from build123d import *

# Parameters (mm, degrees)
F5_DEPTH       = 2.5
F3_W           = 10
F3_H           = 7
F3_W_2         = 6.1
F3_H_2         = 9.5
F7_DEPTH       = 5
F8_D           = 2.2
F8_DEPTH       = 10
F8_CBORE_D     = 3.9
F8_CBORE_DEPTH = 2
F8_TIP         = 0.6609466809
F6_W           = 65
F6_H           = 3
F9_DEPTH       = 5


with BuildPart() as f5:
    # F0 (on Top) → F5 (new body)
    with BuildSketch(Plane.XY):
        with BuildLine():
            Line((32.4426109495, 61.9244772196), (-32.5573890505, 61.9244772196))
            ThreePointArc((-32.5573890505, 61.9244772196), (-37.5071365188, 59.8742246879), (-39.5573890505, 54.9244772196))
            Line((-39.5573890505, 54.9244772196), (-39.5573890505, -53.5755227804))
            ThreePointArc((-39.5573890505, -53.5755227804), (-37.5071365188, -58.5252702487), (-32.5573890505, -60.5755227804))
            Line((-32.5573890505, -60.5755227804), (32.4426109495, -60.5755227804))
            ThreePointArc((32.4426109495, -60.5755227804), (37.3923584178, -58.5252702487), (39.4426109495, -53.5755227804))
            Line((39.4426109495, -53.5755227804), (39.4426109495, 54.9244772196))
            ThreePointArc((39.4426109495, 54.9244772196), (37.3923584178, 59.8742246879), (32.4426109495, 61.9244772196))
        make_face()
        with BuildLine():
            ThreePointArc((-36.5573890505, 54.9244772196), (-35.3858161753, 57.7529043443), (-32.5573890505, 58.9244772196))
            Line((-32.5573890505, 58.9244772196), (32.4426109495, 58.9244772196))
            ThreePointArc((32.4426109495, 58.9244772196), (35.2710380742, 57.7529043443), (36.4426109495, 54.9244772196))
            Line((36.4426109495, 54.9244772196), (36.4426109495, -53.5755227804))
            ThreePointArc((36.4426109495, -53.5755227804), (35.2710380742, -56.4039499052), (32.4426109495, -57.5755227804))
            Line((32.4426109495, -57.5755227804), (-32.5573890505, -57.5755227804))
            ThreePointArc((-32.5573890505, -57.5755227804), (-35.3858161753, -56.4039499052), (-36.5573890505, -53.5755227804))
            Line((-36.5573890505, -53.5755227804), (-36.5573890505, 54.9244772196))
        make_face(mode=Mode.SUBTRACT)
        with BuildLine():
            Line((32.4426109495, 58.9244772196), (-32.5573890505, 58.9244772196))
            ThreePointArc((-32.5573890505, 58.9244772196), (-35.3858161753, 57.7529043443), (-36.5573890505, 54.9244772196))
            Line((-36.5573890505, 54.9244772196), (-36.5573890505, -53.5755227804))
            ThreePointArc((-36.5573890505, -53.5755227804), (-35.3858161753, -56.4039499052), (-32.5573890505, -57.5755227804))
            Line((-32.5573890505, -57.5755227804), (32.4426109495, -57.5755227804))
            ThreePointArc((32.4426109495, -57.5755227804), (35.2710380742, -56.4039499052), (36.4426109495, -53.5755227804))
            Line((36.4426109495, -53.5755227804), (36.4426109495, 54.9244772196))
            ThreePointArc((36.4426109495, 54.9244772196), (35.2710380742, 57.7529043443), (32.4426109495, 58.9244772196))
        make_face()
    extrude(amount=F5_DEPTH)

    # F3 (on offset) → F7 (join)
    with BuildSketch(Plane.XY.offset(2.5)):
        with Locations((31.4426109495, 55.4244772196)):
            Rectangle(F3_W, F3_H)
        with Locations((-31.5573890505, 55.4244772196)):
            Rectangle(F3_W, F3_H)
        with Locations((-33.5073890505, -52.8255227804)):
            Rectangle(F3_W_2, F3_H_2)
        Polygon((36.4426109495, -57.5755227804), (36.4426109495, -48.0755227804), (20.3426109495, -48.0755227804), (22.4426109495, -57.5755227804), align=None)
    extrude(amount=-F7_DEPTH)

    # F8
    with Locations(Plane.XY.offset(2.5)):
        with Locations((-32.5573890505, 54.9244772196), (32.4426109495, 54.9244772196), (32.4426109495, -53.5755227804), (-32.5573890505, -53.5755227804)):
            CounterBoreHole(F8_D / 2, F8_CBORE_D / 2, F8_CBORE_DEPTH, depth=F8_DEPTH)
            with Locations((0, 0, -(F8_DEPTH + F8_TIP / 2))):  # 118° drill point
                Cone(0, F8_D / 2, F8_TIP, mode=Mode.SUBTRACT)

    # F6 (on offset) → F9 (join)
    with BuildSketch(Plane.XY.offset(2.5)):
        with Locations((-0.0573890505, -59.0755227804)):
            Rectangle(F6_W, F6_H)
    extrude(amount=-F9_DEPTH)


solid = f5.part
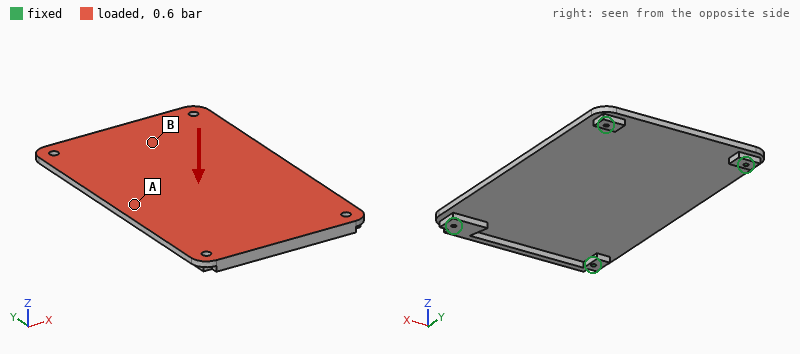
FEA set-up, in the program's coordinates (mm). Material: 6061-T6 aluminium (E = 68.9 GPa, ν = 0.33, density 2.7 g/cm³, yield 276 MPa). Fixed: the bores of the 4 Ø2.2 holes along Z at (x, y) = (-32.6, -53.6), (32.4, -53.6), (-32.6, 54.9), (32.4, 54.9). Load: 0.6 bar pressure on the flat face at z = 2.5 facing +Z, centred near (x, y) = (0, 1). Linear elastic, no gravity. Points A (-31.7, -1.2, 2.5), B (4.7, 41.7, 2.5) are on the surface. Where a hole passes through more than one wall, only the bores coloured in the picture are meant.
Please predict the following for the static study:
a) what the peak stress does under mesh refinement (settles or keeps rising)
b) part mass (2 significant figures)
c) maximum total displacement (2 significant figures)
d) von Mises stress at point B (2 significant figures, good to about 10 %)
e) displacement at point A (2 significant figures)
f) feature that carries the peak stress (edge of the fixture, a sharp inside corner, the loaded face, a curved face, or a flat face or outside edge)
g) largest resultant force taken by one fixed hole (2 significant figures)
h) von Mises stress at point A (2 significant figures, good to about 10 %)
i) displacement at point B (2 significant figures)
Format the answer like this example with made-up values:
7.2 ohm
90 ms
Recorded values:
keeps rising
68 g
0.30 mm
15 MPa
0.29 mm
edge of the fixture
420 N
34 MPa
0.12 mm
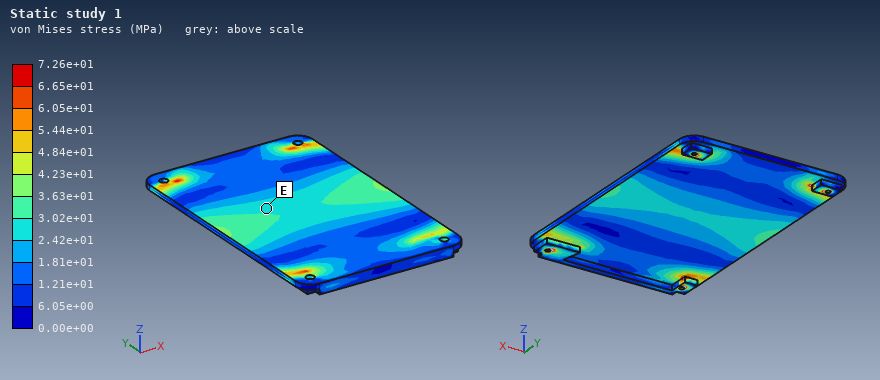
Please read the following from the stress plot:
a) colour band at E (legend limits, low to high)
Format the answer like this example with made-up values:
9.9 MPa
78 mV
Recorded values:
2.42e+01 to 3.02e+01 MPa
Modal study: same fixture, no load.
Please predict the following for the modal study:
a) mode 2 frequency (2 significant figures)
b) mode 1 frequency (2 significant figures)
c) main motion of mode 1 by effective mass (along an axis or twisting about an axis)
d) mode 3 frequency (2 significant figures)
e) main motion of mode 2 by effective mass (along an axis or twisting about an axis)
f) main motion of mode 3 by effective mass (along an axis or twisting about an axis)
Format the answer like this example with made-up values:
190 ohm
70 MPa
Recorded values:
1500 Hz
990 Hz
along Z
2500 Hz
twisting about Y
twisting about X
